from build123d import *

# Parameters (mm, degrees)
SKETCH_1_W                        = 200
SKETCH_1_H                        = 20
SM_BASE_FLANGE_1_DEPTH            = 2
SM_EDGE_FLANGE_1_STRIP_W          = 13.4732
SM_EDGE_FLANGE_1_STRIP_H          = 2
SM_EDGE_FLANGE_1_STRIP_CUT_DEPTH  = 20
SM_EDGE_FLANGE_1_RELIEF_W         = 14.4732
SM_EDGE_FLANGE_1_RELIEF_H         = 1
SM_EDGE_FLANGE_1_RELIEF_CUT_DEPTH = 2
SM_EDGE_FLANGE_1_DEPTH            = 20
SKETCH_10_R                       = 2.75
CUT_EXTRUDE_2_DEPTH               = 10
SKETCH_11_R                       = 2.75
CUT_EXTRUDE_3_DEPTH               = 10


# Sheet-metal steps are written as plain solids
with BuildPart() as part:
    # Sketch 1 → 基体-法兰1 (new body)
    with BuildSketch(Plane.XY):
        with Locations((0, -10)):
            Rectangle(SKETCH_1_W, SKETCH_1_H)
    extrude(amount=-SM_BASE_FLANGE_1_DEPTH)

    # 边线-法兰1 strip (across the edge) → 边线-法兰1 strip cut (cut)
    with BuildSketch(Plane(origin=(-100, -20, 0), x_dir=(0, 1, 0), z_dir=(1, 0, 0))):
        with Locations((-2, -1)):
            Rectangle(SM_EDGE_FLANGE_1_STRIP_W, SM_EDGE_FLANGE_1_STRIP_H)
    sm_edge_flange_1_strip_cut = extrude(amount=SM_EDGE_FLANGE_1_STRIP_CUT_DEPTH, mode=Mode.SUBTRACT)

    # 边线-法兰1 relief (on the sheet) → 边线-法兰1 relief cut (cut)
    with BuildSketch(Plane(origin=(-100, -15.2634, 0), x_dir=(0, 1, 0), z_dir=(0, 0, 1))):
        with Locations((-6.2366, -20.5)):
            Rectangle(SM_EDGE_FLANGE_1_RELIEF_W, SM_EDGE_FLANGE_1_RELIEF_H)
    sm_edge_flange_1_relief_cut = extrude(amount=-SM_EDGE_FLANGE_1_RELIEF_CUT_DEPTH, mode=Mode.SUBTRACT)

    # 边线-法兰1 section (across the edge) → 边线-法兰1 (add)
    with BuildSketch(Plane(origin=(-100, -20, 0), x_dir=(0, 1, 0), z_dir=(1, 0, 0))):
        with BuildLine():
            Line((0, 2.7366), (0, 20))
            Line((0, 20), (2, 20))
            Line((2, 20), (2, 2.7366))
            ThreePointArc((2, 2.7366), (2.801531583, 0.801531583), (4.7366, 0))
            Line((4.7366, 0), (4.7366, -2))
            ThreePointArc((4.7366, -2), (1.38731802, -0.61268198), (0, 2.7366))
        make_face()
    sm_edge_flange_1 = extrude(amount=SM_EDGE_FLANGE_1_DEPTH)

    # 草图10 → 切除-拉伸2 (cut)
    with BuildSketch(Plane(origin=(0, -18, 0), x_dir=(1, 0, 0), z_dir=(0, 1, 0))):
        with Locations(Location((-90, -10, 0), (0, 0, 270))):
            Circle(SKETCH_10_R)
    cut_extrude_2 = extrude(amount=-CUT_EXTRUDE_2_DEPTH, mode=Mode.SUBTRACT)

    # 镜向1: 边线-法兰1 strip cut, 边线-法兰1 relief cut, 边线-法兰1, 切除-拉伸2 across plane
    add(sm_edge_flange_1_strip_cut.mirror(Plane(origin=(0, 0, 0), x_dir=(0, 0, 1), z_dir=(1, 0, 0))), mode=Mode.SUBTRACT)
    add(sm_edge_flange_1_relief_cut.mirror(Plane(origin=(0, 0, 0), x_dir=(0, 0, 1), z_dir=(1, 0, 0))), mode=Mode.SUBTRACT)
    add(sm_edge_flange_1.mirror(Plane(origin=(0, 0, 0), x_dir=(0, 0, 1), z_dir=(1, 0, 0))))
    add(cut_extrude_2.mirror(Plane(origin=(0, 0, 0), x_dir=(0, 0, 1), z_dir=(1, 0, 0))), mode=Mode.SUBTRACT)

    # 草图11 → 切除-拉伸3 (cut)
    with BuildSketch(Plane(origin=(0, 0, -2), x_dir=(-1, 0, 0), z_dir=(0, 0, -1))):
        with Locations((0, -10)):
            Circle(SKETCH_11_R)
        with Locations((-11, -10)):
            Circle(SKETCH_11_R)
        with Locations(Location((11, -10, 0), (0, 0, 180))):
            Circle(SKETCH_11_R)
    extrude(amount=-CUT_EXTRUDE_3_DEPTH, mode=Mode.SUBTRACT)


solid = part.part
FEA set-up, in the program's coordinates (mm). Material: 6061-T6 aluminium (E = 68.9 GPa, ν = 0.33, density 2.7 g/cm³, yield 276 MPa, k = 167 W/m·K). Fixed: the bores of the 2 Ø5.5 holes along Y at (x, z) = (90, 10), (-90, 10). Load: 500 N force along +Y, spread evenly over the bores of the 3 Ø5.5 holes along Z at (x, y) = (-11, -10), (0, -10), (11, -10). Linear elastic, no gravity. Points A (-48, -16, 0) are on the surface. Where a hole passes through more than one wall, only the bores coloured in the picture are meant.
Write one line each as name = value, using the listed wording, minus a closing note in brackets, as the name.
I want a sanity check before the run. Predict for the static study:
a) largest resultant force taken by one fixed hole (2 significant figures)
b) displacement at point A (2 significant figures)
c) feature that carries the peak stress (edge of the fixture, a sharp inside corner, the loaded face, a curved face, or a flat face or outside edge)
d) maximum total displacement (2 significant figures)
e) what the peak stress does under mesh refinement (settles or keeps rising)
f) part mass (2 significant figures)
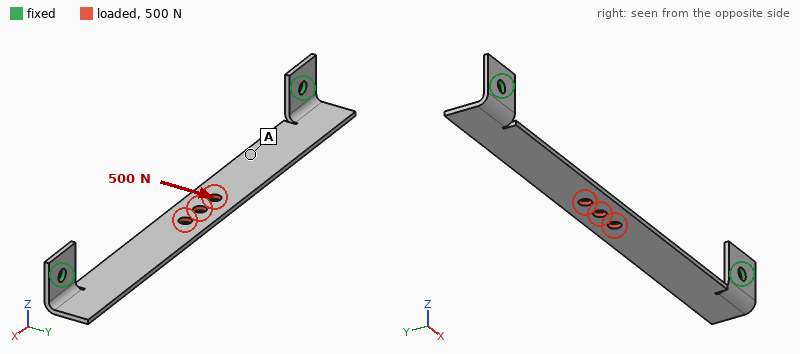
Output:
largest resultant force taken by one fixed hole = 570 N
displacement at point A = 0.36 mm
feature that carries the peak stress = edge of the fixture
maximum total displacement = 0.67 mm
what the peak stress does under mesh refinement = keeps rising
part mass = 25 g
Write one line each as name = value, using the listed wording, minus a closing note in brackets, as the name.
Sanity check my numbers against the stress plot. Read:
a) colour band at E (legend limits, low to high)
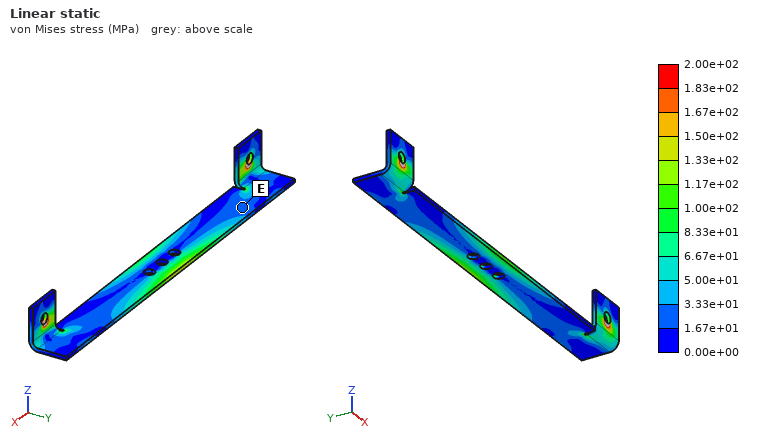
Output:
colour band at E = 1.67e+01 to 3.33e+01 MPa
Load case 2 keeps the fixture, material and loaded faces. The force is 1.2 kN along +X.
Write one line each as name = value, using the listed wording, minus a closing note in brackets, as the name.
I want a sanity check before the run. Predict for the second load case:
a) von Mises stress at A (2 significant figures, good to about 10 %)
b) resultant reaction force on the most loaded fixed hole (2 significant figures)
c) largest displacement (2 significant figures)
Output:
von Mises stress at A = 29 MPa
resultant reaction force on the most loaded fixed hole = 600 N
largest displacement = 92 µm
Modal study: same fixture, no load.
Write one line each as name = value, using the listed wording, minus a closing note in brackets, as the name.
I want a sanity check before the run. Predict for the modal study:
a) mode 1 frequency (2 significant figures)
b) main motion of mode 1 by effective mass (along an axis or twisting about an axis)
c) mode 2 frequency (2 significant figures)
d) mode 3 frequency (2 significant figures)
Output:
mode 1 frequency = 310 Hz
main motion of mode 1 by effective mass = along Z
mode 2 frequency = 860 Hz
mode 3 frequency = 1200 Hz
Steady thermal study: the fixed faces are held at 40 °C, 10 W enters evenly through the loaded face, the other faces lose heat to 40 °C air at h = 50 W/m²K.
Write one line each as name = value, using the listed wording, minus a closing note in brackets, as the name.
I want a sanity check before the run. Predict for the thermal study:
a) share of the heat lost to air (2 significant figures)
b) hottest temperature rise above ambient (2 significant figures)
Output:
share of the heat lost to air = 71 %
hottest temperature rise above ambient = 37 K
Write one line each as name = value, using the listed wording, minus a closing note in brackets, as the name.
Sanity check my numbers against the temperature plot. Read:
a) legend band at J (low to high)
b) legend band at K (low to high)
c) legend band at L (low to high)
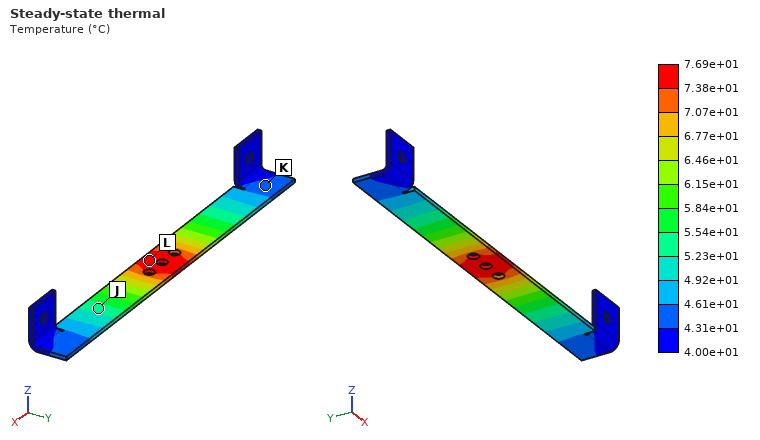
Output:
legend band at J = 5.23e+01 to 5.54e+01 °C
legend band at K = 4.31e+01 to 4.61e+01 °C
legend band at L = 7.38e+01 to 7.69e+01 °C
